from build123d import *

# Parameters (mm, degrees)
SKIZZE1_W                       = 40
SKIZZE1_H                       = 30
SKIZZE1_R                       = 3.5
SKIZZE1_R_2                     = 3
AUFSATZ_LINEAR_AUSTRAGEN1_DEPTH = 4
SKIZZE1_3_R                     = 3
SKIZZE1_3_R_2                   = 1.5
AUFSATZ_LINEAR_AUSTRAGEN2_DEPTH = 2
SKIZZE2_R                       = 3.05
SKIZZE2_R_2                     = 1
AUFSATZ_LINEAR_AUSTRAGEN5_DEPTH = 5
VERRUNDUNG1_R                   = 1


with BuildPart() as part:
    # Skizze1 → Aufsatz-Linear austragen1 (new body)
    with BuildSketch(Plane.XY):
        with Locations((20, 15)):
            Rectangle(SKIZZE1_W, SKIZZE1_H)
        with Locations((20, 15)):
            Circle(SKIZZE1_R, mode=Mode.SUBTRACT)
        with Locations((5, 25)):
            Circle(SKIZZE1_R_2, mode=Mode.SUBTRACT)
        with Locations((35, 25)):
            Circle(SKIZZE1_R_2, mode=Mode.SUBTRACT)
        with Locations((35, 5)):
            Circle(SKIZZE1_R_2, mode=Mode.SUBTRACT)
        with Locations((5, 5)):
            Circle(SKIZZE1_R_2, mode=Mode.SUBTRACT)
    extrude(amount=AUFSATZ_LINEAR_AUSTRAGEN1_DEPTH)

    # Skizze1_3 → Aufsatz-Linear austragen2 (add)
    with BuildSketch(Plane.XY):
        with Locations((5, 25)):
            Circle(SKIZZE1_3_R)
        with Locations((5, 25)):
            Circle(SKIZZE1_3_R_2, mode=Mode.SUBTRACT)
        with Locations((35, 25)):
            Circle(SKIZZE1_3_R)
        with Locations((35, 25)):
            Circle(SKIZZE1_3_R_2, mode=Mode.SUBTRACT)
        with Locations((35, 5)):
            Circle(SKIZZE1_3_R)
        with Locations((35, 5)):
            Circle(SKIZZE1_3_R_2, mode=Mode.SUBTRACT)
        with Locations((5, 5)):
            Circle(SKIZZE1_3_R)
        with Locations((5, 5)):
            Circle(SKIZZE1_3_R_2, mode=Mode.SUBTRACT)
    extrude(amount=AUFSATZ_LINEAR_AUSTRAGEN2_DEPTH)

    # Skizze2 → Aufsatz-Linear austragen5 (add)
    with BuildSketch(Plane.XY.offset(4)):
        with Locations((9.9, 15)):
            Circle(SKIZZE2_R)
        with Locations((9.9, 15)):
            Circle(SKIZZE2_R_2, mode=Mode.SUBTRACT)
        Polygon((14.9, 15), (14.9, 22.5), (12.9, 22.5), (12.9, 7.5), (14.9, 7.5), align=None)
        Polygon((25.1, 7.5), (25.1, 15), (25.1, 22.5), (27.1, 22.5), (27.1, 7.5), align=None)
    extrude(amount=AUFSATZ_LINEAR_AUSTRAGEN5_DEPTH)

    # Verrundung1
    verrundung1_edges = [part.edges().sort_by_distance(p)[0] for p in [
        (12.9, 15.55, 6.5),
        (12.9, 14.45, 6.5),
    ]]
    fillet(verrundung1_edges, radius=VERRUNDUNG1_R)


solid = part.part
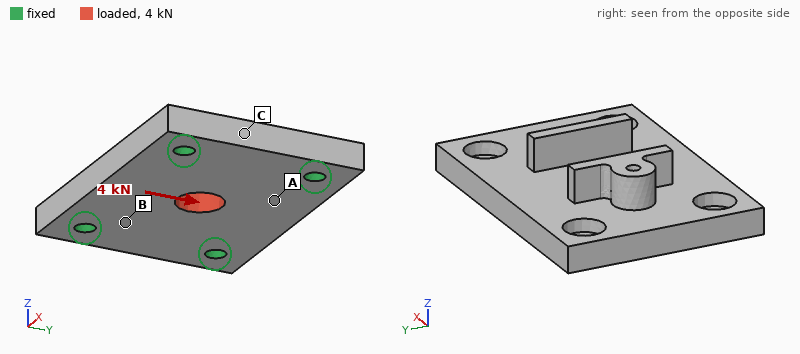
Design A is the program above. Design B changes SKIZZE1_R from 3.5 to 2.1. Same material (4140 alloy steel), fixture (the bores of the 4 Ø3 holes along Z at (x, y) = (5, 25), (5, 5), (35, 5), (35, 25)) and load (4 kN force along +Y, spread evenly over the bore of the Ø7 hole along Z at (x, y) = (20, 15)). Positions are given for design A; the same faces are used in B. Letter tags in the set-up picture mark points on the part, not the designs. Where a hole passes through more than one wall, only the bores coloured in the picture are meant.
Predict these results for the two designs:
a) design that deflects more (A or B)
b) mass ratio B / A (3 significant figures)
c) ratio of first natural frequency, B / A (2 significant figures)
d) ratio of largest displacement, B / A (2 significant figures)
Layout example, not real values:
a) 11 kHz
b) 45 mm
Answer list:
a) B
b) 1.02
c) 1.0
d) 1.1
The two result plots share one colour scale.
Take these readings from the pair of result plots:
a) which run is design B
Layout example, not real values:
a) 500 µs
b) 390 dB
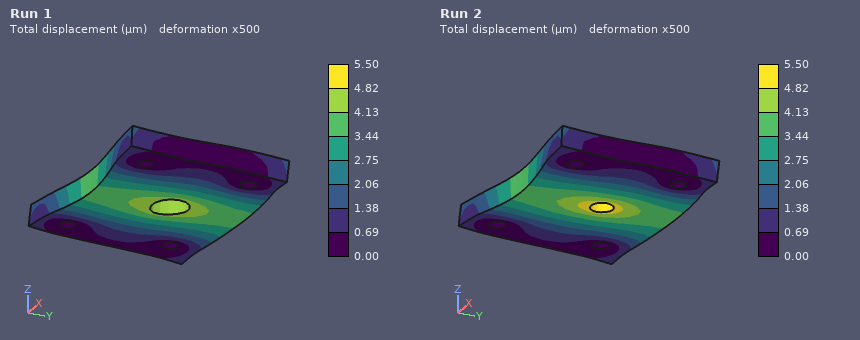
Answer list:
a) Run 2
